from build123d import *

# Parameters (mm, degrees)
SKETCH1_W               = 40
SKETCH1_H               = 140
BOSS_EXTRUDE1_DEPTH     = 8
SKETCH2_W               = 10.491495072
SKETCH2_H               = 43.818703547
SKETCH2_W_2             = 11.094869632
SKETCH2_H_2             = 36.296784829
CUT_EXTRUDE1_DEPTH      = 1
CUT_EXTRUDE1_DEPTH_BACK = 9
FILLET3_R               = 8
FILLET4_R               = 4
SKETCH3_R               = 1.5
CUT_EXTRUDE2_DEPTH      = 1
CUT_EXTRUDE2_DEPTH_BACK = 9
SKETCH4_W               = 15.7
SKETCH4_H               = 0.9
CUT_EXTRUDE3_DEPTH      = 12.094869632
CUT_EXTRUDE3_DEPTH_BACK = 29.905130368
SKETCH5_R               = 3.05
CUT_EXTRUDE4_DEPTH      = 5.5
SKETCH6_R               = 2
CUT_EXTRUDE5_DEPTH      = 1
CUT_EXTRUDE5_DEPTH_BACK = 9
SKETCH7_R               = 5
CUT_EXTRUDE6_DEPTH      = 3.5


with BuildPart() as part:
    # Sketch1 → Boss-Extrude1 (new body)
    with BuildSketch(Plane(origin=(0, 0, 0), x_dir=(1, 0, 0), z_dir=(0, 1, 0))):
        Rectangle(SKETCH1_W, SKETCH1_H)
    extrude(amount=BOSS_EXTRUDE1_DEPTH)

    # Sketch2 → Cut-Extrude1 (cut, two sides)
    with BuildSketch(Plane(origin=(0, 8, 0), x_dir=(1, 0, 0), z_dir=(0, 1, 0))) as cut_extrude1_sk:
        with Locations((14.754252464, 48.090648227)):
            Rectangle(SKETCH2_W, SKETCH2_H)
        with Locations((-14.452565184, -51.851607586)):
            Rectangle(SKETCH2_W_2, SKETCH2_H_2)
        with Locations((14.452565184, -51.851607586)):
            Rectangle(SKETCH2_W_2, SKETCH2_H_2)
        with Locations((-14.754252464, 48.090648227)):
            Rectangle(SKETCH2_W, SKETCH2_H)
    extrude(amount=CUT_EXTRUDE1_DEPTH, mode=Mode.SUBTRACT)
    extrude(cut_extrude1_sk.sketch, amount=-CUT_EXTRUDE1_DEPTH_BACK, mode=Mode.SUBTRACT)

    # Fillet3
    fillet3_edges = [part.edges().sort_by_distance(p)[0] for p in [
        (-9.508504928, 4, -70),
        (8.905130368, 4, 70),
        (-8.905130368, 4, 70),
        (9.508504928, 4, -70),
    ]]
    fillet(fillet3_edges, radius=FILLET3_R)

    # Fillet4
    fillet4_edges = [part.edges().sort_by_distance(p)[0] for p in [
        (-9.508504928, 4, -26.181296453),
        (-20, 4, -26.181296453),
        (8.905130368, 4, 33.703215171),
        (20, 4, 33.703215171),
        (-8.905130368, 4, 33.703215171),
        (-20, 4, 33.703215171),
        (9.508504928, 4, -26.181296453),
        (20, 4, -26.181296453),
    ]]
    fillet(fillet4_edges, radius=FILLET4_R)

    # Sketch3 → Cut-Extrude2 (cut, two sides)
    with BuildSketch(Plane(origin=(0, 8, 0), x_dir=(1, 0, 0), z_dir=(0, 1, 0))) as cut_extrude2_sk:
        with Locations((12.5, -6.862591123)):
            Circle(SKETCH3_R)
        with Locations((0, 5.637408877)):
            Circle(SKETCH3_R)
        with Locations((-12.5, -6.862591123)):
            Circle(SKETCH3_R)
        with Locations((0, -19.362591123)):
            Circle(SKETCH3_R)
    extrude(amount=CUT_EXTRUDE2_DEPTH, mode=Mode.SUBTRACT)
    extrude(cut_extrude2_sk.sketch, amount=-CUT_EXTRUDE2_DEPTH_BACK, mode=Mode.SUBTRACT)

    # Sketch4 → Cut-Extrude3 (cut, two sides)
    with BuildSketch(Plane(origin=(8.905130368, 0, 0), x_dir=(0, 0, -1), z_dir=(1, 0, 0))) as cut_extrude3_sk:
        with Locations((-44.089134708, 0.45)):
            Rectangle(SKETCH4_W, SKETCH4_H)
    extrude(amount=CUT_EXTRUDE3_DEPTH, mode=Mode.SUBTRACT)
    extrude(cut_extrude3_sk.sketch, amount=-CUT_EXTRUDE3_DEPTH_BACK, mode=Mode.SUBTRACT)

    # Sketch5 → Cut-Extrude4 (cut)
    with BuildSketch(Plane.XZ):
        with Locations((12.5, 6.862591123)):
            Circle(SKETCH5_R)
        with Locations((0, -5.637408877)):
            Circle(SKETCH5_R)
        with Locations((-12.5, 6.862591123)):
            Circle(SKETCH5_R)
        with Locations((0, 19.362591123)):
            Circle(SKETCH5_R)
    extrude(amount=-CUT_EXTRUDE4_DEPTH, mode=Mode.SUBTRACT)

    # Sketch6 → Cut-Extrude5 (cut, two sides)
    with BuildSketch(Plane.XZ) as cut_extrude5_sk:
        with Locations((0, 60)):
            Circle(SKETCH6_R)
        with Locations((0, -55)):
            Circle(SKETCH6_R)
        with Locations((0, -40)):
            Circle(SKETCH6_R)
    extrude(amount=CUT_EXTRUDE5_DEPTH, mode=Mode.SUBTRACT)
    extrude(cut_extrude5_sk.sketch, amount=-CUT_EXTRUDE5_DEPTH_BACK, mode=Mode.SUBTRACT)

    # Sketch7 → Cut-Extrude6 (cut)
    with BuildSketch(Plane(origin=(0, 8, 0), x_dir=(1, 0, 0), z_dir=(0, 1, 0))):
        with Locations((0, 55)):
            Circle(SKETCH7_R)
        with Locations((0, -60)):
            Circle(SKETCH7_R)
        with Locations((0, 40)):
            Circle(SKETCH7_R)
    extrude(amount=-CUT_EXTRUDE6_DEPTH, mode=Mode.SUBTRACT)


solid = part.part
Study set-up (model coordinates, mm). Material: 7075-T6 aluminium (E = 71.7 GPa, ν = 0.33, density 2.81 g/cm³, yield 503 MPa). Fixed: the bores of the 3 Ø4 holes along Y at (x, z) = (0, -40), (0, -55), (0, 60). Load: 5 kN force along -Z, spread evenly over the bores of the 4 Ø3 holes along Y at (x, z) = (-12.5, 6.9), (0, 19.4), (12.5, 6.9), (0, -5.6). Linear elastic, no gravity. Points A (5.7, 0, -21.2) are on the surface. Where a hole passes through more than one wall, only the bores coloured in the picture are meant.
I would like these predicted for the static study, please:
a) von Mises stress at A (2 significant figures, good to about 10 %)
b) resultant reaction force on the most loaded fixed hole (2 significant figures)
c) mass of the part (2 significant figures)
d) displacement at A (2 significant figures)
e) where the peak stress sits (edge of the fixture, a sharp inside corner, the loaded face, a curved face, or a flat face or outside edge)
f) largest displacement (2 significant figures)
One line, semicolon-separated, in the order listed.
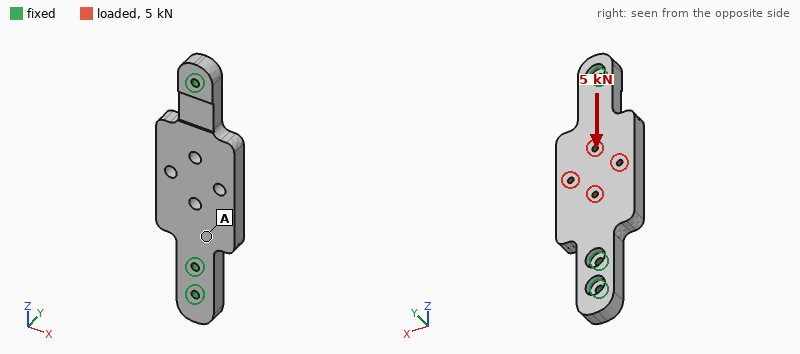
13 MPa; 2.2 kN; 80 g; 6.5 µm; the loaded face; 17 µm
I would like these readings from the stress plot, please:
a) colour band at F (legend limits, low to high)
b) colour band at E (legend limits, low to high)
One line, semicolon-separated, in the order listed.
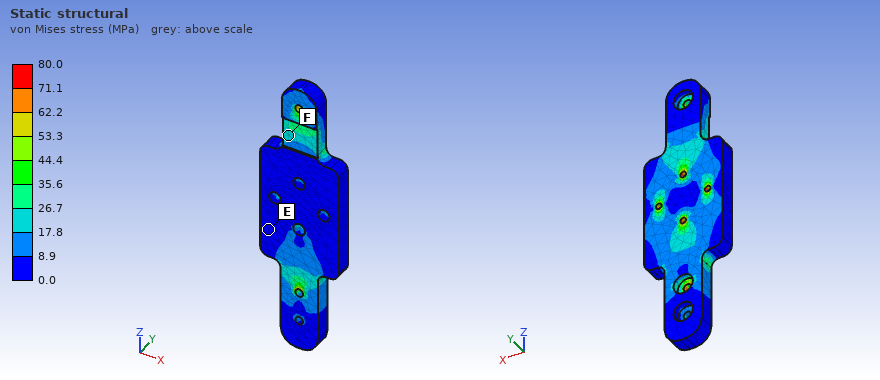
17.8 to 26.7 MPa; 0.0 to 8.9 MPa
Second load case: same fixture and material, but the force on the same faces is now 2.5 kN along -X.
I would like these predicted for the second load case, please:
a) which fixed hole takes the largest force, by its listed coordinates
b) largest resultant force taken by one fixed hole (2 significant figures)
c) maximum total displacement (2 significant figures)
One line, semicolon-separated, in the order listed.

(0, -40); 1.9 kN; 74 µm
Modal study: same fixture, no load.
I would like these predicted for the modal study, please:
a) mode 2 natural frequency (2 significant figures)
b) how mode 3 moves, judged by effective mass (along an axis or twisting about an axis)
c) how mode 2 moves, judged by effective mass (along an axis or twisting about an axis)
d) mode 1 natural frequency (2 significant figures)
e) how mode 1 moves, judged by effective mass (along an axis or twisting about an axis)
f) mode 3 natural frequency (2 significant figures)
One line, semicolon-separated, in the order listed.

3400 Hz; along X; twisting about Z; 2700 Hz; along Y; 6100 Hz
